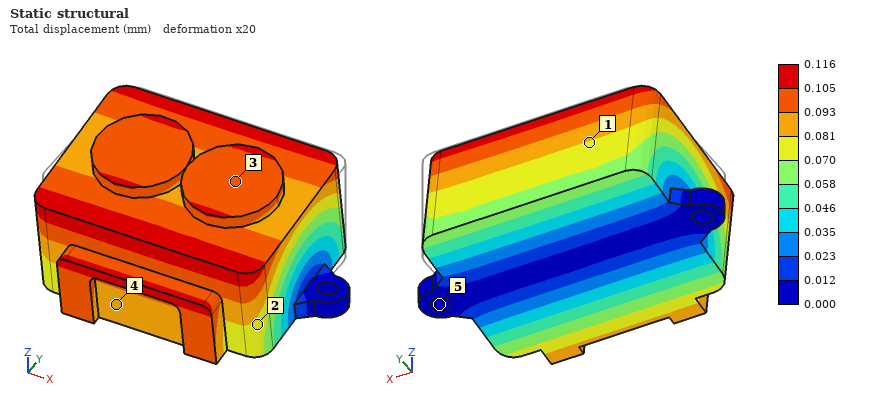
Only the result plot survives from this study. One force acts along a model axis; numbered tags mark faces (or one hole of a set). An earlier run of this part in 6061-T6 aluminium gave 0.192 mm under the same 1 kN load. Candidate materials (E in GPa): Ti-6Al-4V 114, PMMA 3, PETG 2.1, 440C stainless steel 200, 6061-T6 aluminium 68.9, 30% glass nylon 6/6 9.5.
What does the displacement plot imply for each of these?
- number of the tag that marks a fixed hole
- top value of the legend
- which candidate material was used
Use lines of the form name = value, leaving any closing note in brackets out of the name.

number of the tag that marks a fixed hole = 5
top value of the legend = 0.116 mm
which candidate material was used = Ti-6Al-4V
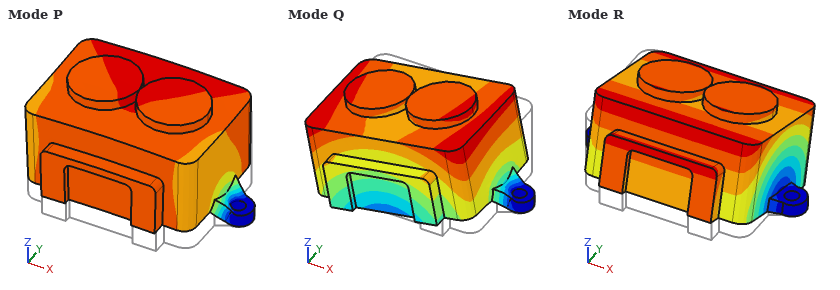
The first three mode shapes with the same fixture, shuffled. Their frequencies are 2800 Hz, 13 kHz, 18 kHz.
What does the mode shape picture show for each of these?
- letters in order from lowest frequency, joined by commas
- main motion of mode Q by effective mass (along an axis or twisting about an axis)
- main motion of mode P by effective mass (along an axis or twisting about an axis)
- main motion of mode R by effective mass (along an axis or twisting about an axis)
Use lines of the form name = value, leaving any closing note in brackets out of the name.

letters in order from lowest frequency, joined by commas = R, P, Q
main motion of mode Q by effective mass = along X
main motion of mode P by effective mass = along Z
main motion of mode R by effective mass = along Y
